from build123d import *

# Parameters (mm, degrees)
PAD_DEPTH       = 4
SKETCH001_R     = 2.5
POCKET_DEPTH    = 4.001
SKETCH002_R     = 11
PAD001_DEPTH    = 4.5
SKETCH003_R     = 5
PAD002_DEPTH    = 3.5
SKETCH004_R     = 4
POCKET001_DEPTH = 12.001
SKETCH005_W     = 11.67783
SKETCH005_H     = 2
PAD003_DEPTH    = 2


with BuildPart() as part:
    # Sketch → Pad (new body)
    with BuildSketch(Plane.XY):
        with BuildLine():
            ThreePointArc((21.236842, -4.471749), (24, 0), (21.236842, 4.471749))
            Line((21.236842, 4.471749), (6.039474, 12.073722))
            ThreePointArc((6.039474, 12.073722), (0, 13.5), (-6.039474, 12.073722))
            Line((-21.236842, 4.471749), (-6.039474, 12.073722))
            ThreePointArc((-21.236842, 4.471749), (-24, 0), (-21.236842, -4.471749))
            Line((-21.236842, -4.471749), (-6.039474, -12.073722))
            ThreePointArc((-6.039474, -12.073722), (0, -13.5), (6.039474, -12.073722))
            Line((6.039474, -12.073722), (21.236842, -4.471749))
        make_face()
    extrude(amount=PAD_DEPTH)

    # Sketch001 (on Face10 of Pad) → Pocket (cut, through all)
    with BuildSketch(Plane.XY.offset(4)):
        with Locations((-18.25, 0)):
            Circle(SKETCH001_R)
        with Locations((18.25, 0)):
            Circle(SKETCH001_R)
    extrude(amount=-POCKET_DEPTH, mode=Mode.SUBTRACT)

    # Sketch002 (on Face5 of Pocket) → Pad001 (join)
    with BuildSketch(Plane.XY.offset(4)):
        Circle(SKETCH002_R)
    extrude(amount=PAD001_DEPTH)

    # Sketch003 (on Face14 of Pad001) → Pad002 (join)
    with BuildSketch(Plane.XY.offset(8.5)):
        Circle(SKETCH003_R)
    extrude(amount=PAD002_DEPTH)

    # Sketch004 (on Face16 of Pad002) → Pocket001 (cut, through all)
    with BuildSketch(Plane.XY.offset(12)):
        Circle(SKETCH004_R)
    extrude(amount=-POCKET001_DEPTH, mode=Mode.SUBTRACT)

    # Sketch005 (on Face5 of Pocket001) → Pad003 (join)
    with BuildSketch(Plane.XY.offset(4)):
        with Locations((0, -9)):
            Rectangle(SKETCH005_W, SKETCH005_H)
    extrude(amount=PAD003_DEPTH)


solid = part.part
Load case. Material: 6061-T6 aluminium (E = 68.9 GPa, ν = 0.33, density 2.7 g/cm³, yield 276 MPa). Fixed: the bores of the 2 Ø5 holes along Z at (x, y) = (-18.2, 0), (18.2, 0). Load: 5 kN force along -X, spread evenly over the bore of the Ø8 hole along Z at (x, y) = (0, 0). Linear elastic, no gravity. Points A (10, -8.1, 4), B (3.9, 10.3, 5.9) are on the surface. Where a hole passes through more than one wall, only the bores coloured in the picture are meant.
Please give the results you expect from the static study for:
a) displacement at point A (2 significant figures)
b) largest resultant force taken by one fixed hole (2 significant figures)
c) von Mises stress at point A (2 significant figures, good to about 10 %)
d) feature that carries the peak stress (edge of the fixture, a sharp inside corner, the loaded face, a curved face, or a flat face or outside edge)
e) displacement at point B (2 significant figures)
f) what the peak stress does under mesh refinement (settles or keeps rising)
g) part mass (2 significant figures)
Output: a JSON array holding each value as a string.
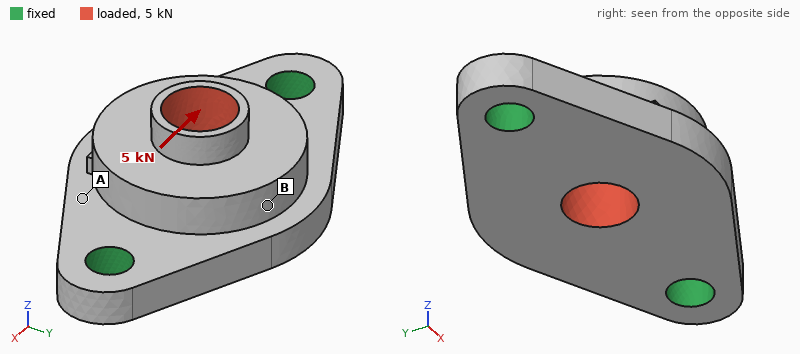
["8.7 µm", "2.6 kN", "38 MPa", "edge of the fixture", "9.7 µm", "keeps rising", "13 g"]
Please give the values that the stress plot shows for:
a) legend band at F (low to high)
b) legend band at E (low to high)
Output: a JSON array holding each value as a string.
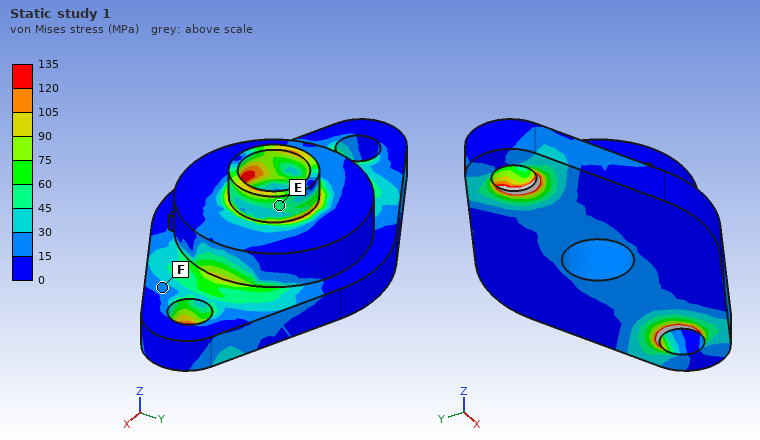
["15 to 30 MPa", "45 to 60 MPa"]
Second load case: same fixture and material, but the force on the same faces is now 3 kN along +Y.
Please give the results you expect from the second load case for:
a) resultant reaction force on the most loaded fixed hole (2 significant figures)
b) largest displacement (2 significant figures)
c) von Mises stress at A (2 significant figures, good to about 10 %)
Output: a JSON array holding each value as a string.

["1.5 kN", "78 µm", "47 MPa"]
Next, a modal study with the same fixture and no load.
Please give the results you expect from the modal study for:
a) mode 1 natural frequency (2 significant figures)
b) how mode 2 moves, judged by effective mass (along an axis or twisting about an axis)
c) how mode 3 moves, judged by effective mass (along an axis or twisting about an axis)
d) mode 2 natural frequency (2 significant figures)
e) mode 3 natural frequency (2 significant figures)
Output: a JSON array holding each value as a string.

["11 kHz", "along Z", "along Y", "15 kHz", "27 kHz"]
